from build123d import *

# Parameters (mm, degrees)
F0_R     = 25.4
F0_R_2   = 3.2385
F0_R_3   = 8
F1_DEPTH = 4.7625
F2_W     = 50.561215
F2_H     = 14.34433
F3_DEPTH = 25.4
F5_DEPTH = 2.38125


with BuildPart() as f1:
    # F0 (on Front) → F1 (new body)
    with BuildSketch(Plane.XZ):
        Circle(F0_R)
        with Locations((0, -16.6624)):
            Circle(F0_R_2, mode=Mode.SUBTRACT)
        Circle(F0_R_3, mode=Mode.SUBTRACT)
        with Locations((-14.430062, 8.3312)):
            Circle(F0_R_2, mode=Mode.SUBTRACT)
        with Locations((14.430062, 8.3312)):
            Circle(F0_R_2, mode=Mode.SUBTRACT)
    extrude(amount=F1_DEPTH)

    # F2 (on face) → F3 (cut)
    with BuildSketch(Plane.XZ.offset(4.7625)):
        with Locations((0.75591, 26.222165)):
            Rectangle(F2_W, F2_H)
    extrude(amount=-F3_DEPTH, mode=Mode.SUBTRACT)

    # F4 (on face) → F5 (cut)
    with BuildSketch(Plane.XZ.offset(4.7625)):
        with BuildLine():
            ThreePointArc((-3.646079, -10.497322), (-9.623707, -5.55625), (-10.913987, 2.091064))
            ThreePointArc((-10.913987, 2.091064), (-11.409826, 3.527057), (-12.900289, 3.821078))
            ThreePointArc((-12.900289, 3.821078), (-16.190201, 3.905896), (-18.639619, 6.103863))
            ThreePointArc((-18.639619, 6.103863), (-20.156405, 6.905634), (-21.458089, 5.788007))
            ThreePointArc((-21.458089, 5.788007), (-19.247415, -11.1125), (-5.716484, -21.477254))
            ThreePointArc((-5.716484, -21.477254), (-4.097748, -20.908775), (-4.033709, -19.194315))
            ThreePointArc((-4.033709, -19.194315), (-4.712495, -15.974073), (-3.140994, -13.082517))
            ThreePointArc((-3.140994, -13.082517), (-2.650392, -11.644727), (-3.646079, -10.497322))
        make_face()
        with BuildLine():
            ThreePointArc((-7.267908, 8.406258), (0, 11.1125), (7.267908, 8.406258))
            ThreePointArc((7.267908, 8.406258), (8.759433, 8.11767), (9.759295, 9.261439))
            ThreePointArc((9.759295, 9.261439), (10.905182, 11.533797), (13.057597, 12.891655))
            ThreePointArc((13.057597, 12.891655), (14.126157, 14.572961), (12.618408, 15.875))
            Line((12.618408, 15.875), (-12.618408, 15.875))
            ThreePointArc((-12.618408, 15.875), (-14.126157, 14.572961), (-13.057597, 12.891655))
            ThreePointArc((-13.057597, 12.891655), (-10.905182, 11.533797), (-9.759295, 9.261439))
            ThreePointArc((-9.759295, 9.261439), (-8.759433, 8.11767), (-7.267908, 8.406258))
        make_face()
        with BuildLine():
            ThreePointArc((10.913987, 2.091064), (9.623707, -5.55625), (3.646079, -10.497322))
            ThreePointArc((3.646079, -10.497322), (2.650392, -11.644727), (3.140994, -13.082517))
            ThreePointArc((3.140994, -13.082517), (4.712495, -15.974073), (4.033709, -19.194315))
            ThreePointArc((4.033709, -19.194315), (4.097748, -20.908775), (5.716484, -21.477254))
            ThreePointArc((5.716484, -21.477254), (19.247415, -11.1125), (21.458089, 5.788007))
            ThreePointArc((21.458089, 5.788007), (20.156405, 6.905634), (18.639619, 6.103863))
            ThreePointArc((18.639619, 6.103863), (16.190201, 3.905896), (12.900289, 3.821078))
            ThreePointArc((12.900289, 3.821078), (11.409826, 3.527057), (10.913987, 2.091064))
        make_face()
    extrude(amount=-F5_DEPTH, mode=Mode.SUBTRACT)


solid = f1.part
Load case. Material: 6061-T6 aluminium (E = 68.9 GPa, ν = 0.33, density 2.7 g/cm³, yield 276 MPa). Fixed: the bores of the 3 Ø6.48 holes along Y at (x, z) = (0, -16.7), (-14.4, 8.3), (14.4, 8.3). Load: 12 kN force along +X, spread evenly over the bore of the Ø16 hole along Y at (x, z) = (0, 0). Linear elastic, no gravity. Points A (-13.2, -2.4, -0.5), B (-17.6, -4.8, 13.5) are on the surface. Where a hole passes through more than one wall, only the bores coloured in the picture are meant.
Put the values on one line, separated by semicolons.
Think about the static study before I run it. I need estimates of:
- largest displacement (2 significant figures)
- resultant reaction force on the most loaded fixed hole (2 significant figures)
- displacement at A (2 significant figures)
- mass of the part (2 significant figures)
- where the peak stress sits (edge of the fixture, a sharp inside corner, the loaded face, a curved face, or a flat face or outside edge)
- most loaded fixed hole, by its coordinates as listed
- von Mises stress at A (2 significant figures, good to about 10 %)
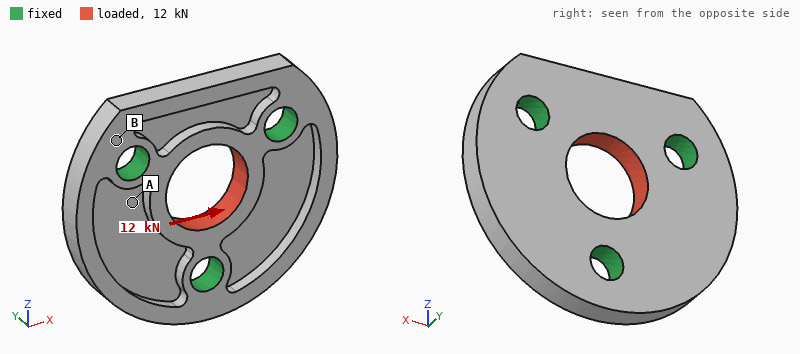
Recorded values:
33 µm; 4.3 kN; 14 µm; 16 g; edge of the fixture; (0, -16.7); 96 MPa
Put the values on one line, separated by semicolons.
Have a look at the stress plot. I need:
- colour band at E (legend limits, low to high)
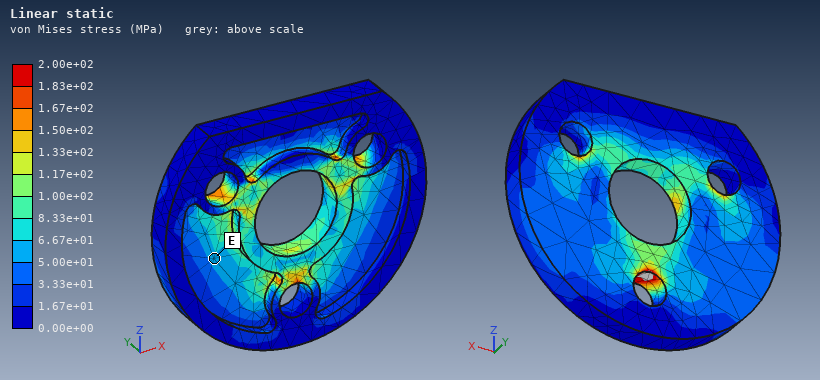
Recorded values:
5.00e+01 to 6.67e+01 MPa
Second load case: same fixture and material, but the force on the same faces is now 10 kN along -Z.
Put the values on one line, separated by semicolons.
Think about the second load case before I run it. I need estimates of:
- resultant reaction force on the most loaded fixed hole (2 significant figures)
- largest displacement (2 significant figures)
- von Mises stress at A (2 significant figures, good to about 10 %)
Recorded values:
3.5 kN; 34 µm; 54 MPa
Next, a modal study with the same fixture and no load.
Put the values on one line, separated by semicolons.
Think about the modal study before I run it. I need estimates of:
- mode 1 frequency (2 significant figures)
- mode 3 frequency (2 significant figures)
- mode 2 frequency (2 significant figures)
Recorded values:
11 kHz; 21 kHz; 11 kHz
